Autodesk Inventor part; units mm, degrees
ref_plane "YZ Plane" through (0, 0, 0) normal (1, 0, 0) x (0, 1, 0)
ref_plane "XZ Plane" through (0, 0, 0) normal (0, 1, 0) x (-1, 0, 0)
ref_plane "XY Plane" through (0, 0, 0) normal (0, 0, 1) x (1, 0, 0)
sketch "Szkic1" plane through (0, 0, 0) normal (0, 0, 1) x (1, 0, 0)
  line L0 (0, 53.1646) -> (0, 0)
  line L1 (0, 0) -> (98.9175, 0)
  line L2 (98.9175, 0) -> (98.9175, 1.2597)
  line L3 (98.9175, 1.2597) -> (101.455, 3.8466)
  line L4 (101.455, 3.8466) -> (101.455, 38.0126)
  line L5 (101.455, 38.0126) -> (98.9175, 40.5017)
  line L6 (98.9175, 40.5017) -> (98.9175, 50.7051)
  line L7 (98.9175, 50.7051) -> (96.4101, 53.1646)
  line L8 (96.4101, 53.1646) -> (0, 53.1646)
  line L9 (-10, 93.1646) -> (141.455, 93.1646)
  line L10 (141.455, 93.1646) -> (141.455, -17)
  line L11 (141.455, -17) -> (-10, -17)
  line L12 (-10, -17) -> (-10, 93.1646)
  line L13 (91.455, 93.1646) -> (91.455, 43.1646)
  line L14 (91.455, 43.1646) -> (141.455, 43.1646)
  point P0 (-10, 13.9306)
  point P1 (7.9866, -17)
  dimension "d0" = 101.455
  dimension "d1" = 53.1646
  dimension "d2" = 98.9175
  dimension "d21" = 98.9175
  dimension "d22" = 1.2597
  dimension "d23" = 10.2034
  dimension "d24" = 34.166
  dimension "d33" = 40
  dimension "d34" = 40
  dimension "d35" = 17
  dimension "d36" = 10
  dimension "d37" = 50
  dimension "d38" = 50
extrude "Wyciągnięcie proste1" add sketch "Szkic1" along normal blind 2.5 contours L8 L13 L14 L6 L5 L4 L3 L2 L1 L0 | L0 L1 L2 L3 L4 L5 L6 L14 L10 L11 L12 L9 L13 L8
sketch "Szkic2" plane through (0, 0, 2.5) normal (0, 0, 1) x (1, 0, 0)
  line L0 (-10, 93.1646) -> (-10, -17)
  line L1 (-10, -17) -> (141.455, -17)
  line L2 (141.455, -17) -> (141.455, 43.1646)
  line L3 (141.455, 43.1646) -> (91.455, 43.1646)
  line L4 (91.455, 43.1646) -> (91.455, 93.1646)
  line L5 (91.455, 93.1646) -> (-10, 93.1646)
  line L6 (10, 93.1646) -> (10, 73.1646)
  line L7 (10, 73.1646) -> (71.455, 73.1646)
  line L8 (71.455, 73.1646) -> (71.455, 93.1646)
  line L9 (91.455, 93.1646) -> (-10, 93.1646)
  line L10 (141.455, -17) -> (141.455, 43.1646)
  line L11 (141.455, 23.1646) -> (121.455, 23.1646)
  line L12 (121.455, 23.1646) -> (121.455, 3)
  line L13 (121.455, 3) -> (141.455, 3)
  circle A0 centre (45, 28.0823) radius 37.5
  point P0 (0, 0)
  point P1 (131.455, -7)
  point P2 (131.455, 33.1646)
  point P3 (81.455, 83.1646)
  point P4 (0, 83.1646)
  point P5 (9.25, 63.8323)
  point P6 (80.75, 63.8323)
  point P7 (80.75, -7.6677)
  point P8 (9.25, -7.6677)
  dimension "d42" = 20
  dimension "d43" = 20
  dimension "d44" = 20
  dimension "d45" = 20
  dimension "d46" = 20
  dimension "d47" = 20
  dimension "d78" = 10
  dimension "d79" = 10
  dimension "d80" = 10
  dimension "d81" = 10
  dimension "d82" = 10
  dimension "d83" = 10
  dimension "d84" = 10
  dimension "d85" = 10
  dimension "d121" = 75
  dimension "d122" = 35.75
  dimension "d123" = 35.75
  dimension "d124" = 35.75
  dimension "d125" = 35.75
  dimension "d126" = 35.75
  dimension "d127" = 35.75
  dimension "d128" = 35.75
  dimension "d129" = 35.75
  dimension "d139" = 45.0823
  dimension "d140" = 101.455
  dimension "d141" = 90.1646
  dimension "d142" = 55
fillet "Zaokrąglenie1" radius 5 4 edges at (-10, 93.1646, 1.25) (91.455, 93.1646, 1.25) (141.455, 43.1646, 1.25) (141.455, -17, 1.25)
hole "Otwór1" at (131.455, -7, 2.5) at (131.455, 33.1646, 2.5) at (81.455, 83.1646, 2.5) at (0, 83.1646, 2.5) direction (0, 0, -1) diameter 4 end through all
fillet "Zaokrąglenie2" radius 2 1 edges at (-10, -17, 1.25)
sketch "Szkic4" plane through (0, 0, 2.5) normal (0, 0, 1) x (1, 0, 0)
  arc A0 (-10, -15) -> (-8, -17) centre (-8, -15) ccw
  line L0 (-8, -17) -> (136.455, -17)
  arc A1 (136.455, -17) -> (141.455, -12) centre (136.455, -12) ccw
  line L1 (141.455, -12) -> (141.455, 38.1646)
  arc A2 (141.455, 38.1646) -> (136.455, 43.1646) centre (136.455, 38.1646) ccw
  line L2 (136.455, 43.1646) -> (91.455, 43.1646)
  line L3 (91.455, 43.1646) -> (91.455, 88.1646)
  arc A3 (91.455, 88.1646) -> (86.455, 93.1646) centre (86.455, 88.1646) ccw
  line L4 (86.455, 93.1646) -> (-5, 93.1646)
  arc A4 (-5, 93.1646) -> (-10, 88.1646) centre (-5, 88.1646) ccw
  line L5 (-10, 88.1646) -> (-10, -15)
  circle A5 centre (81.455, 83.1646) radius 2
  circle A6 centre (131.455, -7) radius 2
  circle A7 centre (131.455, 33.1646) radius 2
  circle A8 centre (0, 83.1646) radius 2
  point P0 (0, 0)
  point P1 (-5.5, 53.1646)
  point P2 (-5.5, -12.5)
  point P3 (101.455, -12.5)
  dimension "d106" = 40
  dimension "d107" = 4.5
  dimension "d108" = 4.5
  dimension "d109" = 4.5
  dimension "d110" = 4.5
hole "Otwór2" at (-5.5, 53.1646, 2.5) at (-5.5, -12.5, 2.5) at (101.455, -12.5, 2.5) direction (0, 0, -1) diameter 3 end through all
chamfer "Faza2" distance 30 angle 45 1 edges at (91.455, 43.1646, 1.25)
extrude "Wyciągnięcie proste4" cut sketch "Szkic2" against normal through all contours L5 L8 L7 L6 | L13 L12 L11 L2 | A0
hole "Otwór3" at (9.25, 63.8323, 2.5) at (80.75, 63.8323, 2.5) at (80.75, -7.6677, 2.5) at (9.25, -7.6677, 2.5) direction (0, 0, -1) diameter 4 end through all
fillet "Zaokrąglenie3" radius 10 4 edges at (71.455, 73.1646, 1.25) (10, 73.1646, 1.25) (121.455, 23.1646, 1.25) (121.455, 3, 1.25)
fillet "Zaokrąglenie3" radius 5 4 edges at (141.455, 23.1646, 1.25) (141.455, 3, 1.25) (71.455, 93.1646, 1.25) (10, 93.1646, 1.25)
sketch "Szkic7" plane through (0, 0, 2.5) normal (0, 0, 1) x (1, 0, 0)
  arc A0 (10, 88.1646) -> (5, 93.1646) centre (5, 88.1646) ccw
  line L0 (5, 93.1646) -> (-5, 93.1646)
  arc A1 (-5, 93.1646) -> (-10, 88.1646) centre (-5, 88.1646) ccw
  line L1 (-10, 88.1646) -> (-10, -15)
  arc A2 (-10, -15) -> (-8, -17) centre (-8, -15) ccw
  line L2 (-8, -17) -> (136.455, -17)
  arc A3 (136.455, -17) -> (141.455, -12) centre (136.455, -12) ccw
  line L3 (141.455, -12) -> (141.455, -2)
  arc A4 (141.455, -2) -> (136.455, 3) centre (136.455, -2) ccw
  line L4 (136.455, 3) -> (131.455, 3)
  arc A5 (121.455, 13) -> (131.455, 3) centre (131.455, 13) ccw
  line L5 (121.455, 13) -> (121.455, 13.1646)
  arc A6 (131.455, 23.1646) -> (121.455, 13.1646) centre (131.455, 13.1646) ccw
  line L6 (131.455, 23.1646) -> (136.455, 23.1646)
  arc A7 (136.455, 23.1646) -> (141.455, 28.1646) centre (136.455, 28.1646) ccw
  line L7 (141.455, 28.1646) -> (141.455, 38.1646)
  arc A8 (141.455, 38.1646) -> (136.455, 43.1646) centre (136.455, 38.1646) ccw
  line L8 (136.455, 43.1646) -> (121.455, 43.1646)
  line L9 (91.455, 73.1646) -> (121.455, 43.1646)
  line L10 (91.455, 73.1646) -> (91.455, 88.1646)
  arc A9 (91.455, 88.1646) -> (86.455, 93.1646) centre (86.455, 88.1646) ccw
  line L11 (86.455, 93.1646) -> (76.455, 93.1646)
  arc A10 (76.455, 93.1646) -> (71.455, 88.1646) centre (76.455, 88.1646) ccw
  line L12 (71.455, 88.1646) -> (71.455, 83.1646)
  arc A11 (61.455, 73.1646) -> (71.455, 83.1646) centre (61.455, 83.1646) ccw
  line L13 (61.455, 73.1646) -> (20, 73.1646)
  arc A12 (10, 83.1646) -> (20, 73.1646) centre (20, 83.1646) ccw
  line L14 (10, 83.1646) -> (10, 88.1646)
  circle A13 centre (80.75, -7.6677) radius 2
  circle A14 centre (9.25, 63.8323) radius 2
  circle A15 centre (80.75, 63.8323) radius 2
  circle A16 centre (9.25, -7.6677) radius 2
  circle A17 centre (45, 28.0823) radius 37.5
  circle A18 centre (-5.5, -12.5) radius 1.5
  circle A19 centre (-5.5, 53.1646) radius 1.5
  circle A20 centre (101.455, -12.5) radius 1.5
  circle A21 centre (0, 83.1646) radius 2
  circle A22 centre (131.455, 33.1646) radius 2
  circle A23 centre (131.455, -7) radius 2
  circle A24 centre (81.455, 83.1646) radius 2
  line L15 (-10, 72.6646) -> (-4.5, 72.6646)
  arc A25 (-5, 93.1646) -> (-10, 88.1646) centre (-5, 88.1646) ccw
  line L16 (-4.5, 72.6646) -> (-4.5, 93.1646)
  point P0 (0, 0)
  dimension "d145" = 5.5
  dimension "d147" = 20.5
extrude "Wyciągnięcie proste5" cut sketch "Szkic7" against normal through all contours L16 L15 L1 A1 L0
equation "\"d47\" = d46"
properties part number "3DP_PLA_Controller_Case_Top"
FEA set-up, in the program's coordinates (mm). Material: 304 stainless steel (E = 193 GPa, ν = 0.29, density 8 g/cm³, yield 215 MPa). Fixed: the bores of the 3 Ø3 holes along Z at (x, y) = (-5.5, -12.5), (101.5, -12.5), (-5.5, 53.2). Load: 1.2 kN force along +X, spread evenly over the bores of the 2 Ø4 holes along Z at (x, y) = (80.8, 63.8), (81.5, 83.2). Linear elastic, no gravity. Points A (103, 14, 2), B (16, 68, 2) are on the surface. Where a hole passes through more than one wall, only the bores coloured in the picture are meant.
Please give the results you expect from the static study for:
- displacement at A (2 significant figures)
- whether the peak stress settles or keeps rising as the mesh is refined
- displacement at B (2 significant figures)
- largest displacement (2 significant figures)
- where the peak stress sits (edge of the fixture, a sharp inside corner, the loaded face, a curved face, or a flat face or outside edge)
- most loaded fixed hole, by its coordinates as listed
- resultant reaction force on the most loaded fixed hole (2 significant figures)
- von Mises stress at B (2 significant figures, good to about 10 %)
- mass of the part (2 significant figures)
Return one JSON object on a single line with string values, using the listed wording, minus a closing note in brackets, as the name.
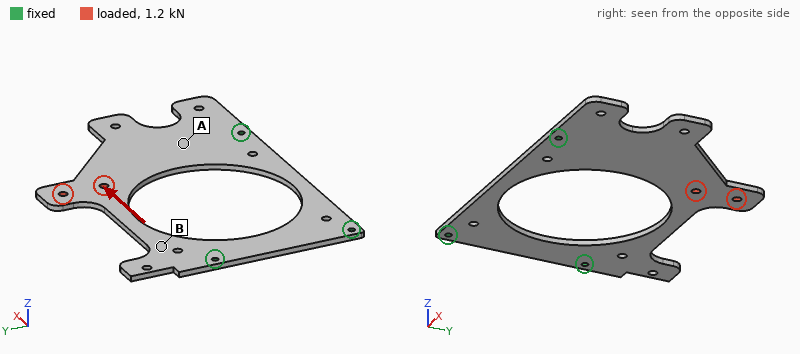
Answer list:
{"displacement at A": "8.7 µm", "whether the peak stress settles or keeps rising as the mesh is refined": "keeps rising", "displacement at B": "14 µm", "largest displacement": "35 µm", "where the peak stress sits": "edge of the fixture", "most loaded fixed hole, by its coordinates as listed": "(-5.5, 53.2)", "resultant reaction force on the most loaded fixed hole": "1.2 kN", "von Mises stress at B": "23 MPa", "mass of the part": "170 g"}
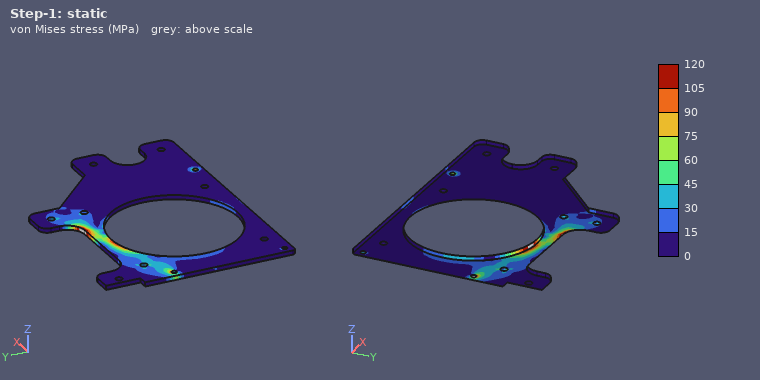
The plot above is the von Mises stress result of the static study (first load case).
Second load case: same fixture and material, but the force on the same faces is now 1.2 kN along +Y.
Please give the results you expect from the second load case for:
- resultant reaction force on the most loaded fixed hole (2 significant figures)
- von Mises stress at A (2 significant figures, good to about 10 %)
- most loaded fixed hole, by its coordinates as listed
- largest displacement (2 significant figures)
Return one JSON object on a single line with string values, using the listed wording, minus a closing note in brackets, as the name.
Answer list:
{"resultant reaction force on the most loaded fixed hole": "1.1 kN", "von Mises stress at A": "15 MPa", "most loaded fixed hole, by its coordinates as listed": "(101.5, -12.5)", "largest displacement": "14 µm"}
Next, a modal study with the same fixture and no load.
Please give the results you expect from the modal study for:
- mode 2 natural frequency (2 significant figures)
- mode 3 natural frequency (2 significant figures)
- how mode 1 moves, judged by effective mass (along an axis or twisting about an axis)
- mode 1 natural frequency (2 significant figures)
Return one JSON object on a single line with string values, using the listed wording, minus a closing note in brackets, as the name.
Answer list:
{"mode 2 natural frequency": "720 Hz", "mode 3 natural frequency": "1200 Hz", "how mode 1 moves, judged by effective mass": "along Z", "mode 1 natural frequency": "290 Hz"}
